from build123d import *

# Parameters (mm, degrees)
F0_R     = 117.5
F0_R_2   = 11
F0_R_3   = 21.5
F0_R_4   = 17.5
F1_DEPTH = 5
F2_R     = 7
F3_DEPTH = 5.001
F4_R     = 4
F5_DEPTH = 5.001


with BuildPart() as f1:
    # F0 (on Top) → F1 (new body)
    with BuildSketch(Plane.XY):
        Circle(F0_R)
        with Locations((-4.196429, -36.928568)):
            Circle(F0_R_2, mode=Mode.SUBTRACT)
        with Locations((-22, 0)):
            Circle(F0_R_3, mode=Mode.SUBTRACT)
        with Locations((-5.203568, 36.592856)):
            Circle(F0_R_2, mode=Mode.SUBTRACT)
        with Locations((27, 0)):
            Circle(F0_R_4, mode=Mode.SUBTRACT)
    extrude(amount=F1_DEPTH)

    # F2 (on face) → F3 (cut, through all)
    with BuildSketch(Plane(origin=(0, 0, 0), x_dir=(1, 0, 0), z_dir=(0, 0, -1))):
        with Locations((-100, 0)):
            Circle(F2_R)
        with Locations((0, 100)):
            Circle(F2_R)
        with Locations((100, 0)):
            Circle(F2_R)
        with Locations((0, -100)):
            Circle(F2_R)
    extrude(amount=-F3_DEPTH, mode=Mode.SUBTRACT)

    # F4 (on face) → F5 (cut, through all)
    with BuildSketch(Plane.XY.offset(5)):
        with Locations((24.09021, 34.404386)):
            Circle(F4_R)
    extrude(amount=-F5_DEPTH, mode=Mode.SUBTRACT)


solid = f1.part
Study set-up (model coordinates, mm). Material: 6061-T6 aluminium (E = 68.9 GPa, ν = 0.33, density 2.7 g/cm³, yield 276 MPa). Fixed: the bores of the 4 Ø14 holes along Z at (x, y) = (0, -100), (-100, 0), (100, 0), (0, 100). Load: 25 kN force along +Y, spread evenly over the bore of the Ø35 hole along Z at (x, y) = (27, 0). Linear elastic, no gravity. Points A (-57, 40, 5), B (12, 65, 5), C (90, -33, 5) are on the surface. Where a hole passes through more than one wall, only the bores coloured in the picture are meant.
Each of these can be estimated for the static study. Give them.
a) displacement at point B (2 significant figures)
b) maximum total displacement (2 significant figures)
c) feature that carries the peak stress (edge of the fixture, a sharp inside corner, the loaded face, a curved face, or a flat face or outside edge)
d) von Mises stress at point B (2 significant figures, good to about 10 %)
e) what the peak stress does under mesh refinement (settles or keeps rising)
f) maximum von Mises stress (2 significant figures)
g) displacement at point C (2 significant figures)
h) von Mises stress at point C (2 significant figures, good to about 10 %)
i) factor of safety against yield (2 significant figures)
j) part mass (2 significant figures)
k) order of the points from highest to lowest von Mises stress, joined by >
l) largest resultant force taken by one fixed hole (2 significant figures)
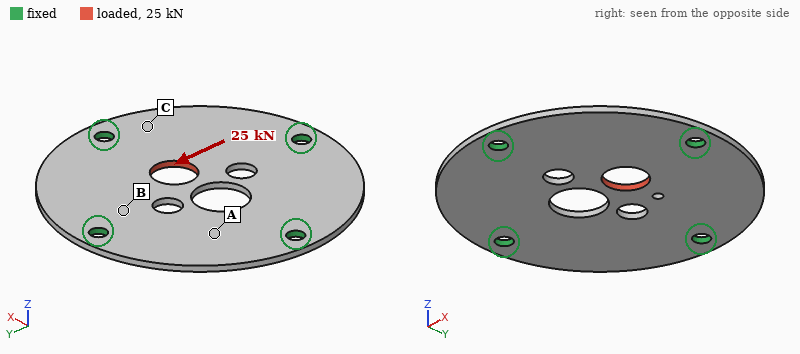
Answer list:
25 µm
63 µm
a curved face
47 MPa
settles
140 MPa
22 µm
22 MPa
1.9
530 g
B > C > A
8.3 kN
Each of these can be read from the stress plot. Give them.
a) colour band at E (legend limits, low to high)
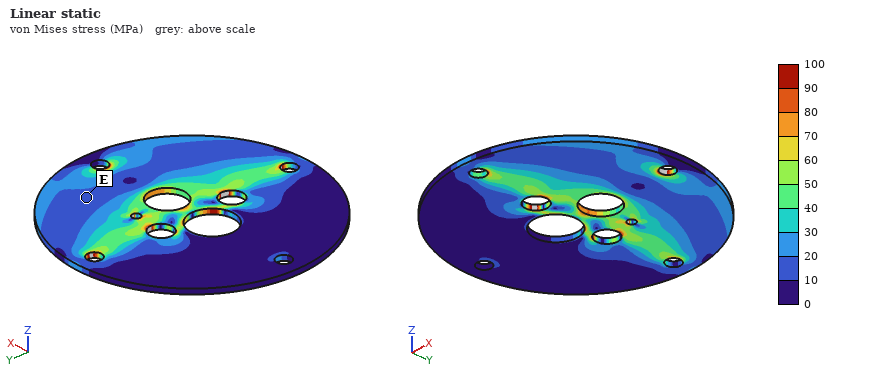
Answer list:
10 to 20 MPa
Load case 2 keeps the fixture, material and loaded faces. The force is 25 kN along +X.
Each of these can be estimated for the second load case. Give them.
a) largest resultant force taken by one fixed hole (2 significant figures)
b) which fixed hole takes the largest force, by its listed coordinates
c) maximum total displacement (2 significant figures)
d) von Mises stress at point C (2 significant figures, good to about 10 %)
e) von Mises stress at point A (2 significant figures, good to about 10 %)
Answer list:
12 kN
(100, 0)
95 µm
15 MPa
16 MPa
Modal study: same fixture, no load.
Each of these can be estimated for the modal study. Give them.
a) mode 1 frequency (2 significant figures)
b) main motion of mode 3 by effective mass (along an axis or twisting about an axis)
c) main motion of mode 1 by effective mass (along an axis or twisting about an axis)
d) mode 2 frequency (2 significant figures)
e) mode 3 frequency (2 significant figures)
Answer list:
1100 Hz
twisting about X
along Z
1100 Hz
1200 Hz
